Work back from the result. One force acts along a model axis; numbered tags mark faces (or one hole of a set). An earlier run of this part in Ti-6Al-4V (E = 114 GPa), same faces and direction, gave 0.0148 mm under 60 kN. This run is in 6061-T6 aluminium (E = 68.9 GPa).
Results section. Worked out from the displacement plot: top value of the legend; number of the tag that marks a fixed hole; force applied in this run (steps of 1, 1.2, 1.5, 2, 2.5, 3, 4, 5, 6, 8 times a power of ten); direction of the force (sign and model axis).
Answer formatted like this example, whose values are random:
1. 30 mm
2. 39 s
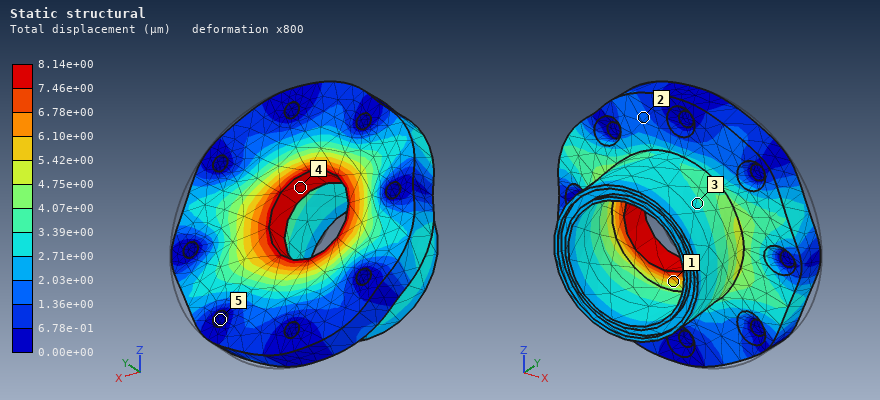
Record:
1. 8.14e+00 µm
2. 5
3. 20 kN
4. -X
